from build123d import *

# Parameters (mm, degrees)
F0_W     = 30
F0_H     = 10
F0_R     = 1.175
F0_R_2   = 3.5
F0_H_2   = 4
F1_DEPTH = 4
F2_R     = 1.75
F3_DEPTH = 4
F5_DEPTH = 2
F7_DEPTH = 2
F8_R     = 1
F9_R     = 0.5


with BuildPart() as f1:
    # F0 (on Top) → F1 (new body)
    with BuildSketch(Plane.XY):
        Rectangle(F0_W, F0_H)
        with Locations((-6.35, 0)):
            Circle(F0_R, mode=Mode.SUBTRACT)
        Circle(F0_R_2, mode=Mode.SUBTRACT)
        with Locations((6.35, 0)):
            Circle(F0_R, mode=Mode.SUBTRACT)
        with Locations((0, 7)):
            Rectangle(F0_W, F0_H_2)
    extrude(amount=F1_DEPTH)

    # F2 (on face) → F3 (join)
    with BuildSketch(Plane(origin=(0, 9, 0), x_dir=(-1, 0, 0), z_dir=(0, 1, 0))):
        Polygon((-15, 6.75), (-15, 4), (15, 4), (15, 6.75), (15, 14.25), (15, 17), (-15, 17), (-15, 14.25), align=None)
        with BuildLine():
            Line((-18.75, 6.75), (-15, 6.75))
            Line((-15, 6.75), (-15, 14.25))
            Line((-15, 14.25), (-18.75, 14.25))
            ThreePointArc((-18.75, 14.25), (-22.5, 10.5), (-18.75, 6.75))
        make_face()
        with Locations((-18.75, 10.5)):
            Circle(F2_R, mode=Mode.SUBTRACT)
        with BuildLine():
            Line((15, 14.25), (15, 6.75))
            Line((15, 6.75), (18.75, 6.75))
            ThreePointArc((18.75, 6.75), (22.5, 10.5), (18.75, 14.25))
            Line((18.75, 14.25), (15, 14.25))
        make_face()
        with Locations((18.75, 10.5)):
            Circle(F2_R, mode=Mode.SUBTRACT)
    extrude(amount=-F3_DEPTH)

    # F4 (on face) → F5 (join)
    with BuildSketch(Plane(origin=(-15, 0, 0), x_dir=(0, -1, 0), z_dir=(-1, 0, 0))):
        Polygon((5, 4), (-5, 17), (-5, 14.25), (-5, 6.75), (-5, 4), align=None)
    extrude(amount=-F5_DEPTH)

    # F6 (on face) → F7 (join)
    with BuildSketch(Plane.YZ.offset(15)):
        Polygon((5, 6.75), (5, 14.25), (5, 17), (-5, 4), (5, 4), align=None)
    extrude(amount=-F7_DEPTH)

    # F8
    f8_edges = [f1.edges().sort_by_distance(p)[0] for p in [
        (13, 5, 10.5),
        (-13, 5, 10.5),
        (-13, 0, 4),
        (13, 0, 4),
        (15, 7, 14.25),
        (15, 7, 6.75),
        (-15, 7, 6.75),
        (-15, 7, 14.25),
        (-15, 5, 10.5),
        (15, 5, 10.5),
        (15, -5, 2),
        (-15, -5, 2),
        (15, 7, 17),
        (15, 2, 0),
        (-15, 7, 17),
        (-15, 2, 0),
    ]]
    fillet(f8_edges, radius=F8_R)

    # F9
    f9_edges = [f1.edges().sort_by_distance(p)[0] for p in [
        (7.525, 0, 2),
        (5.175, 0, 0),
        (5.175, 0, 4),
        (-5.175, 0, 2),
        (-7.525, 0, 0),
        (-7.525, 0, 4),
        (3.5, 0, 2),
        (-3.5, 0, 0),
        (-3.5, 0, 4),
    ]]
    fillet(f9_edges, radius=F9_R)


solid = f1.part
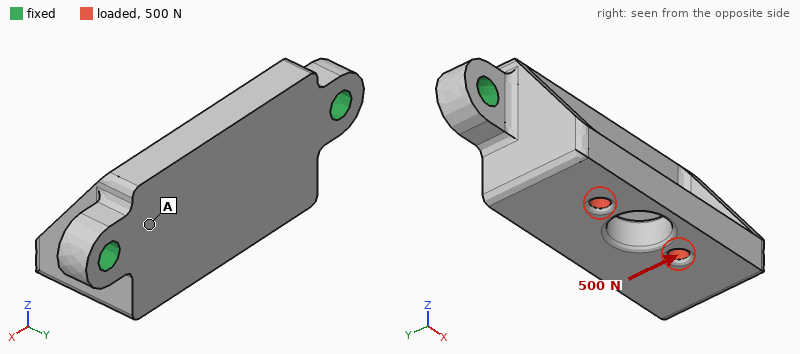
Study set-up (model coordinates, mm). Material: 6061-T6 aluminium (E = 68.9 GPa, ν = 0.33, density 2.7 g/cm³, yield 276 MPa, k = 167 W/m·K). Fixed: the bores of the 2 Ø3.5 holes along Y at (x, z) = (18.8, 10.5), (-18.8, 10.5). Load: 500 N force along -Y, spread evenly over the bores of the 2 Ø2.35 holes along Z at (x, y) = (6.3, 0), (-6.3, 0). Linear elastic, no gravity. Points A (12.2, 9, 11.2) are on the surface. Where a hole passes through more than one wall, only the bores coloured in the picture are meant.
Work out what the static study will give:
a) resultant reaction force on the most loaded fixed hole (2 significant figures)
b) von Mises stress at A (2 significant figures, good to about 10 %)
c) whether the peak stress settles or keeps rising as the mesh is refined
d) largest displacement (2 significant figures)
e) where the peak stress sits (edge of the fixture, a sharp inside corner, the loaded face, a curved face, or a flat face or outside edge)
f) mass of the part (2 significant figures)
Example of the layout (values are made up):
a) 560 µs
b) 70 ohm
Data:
a) 260 N
b) 22 MPa
c) keeps rising
d) 50 µm
e) edge of the fixture
f) 9.8 g
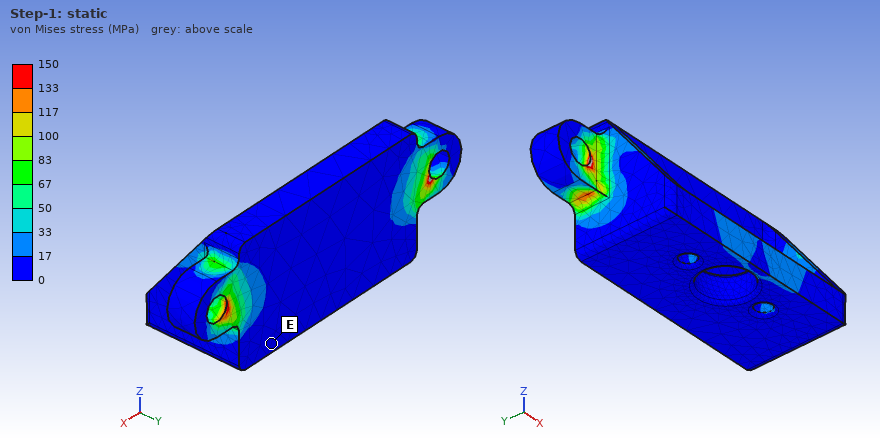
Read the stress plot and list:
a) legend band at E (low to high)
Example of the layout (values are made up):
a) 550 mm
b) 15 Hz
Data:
a) 0 to 17 MPa
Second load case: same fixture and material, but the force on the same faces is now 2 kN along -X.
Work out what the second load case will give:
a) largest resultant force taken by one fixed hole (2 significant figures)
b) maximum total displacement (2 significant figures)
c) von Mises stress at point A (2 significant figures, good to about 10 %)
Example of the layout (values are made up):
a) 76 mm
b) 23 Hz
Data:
a) 1.2 kN
b) 44 µm
c) 14 MPa
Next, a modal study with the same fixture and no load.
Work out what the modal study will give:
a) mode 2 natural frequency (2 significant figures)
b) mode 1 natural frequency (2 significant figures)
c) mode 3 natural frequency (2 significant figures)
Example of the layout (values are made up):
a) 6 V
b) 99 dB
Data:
a) 16 kHz
b) 8100 Hz
c) 16 kHz
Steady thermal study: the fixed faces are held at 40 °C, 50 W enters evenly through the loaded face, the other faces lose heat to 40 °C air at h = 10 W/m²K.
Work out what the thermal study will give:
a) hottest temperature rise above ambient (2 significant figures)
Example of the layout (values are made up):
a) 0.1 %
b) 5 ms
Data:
a) 61 K
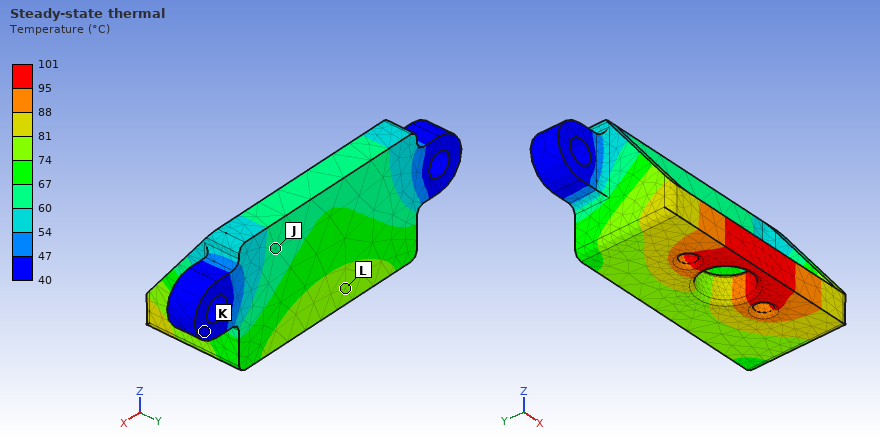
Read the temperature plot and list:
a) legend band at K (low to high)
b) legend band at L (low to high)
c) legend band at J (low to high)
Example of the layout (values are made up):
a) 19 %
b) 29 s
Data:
a) 40 to 47 °C
b) 74 to 81 °C
c) 60 to 67 °C
